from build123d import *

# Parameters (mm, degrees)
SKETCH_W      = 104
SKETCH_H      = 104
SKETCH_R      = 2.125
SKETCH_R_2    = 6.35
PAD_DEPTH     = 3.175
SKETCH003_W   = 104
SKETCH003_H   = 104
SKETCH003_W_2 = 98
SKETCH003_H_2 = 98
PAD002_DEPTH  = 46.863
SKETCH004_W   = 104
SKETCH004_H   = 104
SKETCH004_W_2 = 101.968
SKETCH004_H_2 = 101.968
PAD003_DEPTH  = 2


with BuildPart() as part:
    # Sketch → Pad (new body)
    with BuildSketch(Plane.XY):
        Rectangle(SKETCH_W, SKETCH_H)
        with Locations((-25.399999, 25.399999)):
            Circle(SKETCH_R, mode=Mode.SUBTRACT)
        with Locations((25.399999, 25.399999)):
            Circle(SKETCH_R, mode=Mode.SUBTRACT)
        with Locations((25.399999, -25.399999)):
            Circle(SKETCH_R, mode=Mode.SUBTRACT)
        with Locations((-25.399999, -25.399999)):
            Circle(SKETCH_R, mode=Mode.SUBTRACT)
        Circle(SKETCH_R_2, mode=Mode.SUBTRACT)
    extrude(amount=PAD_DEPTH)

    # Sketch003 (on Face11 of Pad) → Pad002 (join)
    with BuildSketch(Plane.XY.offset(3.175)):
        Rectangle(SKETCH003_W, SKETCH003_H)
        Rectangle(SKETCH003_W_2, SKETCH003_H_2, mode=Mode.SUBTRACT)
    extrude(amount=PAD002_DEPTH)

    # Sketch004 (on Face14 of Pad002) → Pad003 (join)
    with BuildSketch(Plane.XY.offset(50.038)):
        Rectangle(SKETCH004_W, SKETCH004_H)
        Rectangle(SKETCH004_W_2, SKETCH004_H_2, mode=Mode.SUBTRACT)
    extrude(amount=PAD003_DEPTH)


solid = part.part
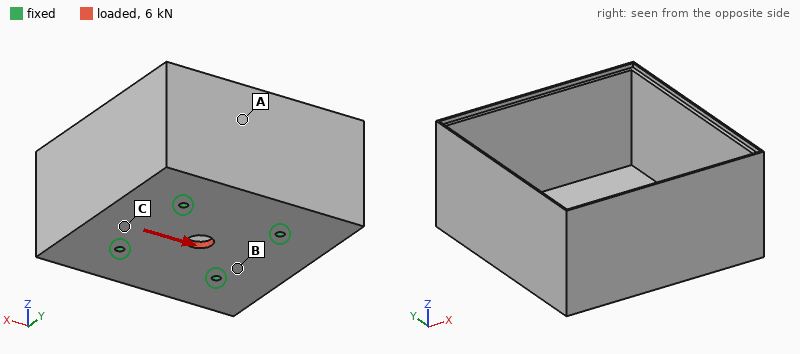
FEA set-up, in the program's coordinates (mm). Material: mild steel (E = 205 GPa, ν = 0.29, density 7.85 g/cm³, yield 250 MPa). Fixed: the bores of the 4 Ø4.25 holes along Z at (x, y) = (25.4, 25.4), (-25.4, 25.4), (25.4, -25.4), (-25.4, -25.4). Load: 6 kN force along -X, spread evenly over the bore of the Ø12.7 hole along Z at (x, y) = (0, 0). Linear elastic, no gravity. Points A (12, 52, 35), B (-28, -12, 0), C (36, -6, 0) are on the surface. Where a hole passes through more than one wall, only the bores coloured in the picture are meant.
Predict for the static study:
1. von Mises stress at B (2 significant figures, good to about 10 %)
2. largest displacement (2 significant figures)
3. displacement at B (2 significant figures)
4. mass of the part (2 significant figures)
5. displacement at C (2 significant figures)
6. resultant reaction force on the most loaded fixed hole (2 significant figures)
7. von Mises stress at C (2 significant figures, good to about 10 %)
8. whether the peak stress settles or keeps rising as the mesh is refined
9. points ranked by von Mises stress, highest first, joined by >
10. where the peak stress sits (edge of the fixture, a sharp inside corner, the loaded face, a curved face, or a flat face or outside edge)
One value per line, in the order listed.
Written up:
14 MPa
5.5 µm
2.1 µm
720 g
2.2 µm
1.6 kN
9.7 MPa
keeps rising
B > C > A
edge of the fixture
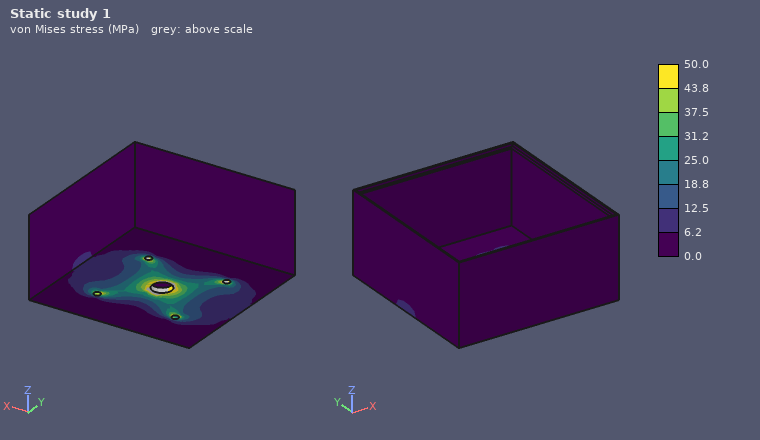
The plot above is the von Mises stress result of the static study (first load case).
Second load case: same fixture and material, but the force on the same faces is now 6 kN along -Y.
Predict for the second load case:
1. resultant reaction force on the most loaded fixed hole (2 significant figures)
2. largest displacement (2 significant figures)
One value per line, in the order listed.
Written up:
1.6 kN
5.5 µm
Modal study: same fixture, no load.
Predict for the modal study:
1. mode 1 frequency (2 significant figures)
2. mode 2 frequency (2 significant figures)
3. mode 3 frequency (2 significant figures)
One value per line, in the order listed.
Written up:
990 Hz
1100 Hz
1100 Hz
